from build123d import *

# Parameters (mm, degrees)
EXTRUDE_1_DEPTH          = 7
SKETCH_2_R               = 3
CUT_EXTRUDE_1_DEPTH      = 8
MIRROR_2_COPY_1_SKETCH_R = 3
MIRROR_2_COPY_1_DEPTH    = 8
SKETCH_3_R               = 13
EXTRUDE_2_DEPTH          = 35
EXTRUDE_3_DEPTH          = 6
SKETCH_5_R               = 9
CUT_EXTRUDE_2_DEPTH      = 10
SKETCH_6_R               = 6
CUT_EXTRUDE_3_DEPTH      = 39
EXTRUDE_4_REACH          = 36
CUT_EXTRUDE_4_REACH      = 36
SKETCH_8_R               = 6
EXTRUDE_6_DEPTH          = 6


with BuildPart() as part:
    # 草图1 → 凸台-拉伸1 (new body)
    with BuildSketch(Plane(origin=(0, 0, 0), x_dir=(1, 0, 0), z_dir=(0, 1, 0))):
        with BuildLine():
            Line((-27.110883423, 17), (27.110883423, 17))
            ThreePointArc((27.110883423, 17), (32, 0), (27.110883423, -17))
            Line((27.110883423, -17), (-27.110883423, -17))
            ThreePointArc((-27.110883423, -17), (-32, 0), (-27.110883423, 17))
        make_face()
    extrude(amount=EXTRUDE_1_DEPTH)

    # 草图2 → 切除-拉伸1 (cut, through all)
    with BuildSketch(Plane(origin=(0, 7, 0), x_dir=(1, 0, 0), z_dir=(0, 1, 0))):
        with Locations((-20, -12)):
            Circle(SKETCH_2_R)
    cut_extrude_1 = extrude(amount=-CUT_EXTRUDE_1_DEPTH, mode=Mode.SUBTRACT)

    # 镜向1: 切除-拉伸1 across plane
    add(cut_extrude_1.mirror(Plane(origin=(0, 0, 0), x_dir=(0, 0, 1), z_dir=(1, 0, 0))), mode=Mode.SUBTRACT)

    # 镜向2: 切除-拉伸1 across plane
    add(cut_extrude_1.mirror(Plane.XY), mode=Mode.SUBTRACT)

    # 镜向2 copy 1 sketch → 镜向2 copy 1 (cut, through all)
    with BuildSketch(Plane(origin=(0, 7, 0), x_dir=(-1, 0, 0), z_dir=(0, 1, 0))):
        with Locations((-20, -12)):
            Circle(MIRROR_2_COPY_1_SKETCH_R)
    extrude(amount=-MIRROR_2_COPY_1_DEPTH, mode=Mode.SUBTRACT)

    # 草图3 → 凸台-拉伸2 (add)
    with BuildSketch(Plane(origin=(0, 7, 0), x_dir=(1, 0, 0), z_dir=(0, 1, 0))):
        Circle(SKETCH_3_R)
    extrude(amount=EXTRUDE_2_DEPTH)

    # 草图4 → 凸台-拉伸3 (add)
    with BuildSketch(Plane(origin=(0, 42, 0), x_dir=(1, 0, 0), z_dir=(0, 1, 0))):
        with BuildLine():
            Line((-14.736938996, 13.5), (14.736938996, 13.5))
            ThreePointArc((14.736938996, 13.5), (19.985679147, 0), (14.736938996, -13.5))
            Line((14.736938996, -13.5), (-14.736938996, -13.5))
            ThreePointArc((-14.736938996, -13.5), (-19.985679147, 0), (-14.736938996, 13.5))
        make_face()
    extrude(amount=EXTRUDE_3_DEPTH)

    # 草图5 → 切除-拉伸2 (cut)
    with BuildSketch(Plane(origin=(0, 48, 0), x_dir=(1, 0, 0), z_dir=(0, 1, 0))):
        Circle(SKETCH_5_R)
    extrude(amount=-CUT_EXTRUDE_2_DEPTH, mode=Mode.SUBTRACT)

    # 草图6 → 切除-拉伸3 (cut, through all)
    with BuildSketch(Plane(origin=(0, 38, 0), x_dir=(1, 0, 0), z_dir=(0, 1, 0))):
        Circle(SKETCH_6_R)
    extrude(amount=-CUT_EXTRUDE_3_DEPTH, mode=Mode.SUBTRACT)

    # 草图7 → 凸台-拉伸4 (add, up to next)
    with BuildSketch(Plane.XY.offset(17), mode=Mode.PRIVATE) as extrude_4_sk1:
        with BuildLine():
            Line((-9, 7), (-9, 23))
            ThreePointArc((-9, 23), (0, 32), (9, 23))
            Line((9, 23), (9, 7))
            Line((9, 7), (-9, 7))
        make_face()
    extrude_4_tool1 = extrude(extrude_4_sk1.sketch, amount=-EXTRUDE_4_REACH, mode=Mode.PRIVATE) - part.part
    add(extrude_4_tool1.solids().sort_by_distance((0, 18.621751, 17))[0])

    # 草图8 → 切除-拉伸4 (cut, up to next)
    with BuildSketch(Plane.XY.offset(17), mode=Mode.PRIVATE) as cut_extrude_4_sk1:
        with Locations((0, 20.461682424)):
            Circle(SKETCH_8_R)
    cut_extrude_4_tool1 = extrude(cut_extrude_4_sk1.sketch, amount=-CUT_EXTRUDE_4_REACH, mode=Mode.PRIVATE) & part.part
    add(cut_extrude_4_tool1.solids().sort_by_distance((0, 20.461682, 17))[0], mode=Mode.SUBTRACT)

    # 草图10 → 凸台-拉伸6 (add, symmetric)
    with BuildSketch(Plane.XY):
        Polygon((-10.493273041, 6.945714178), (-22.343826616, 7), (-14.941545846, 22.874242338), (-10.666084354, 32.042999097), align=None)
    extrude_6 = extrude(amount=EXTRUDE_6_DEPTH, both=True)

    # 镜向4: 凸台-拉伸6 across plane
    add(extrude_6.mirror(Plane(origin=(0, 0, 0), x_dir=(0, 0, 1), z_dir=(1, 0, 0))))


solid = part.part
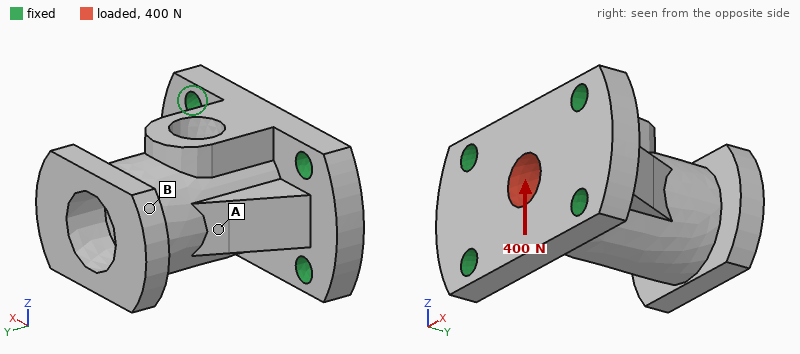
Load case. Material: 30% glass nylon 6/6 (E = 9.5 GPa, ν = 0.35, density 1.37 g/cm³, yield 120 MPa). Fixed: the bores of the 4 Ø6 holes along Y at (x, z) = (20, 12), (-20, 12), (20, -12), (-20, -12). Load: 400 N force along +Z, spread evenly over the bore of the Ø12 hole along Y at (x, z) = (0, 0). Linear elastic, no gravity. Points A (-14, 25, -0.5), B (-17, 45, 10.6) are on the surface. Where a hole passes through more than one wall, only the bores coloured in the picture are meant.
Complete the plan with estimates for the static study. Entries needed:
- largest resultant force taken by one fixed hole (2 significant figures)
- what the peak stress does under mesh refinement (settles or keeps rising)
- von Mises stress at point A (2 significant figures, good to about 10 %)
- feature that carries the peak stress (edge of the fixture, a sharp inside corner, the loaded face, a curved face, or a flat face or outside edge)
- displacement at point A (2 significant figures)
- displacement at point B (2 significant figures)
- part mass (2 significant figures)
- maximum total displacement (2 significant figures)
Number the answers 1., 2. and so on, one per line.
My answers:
1. 190 N
2. keeps rising
3. 1.2 MPa
4. edge of the fixture
5. 17 µm
6. 36 µm
7. 47 g
8. 39 µm
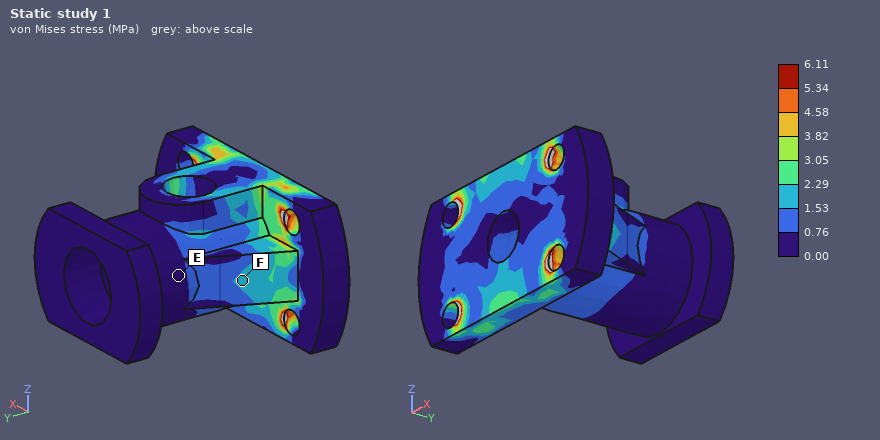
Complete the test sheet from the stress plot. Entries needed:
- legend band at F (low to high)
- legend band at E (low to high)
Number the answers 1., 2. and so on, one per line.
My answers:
1. 1.53 to 2.29 MPa
2. 0.00 to 0.76 MPa
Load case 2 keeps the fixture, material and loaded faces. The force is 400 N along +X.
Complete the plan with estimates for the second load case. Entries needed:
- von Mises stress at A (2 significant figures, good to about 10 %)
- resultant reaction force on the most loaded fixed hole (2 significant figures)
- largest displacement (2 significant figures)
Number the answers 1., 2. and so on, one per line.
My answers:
1. 0.78 MPa
2. 130 N
3. 12 µm
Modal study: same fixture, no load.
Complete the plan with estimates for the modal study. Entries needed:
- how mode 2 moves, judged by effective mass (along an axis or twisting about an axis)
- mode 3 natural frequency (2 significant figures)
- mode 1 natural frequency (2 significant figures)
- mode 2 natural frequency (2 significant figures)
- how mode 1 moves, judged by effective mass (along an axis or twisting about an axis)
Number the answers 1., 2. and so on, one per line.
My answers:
1. along X
2. 7100 Hz
3. 2700 Hz
4. 4500 Hz
5. along Z
